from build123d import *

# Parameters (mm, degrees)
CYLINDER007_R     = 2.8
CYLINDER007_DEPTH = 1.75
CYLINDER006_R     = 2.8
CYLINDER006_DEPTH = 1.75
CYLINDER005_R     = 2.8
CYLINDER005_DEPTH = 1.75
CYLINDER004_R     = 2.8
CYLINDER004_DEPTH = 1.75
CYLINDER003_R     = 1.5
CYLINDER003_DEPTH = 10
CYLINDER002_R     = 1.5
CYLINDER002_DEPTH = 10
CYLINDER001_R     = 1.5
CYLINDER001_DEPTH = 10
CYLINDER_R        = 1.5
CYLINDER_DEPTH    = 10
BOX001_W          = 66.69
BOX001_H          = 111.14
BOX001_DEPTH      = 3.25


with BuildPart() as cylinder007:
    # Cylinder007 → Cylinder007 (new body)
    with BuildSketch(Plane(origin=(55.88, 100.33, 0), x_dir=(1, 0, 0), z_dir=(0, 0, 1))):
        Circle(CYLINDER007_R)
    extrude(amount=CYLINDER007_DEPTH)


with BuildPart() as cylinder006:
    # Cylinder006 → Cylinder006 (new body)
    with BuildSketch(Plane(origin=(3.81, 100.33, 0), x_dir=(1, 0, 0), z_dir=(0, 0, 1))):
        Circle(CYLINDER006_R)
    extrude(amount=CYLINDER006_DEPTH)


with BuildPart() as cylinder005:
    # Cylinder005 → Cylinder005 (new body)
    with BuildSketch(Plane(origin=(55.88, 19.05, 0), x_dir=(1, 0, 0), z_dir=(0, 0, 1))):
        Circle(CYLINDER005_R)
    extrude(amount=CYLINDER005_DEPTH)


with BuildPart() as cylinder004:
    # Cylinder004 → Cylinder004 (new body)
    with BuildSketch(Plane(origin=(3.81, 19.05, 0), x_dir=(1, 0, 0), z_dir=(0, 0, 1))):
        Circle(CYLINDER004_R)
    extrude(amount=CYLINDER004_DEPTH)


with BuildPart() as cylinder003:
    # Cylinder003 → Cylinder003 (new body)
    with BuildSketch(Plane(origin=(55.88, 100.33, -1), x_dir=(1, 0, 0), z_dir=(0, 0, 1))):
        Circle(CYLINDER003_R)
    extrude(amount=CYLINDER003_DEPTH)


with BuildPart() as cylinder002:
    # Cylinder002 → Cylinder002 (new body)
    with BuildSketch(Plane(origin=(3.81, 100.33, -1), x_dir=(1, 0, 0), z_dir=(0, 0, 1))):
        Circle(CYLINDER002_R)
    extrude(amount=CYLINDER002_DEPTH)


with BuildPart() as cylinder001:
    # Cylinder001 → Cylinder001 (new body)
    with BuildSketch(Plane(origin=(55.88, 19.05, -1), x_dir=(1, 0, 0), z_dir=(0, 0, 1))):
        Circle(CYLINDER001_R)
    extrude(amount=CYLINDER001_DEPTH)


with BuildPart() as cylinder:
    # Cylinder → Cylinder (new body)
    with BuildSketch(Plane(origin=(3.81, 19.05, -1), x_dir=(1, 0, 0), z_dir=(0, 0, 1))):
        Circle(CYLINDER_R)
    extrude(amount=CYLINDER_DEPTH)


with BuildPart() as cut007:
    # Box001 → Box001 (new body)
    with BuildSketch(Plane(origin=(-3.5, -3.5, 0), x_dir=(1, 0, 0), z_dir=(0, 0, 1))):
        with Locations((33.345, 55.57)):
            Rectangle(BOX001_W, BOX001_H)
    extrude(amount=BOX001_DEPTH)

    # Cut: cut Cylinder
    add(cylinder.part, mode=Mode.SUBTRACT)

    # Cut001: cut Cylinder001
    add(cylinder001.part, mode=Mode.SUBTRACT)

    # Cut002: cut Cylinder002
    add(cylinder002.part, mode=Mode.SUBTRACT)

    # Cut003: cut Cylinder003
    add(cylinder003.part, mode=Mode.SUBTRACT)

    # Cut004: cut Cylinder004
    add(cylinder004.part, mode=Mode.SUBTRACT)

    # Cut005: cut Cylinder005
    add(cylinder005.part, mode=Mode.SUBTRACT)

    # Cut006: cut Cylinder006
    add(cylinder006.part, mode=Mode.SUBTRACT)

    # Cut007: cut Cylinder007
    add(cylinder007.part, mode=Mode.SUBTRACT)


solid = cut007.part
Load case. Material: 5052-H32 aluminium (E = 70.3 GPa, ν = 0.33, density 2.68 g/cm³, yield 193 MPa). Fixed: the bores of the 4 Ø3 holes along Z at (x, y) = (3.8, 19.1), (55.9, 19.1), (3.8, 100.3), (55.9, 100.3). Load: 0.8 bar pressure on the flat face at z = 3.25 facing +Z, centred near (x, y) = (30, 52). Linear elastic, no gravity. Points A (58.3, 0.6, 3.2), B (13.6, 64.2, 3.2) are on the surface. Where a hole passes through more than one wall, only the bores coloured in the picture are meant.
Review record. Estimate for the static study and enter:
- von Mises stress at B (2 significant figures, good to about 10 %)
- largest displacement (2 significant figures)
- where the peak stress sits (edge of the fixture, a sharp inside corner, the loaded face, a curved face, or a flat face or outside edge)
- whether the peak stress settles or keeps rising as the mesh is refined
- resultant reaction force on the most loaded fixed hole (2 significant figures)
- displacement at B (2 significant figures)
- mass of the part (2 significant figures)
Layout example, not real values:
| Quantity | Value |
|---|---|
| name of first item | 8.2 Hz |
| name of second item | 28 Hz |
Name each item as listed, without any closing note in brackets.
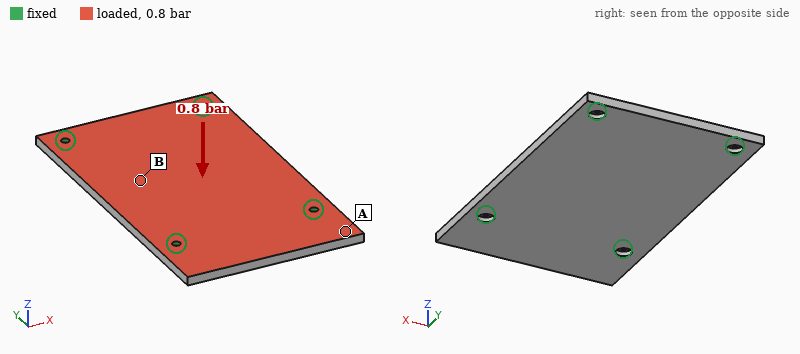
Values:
| Quantity | Value |
|---|---|
| von Mises stress at B | 14 MPa |
| largest displacement | 87 µm |
| where the peak stress sits | edge of the fixture |
| whether the peak stress settles or keeps rising as the mesh is refined | keeps rising |
| resultant reaction force on the most loaded fixed hole | 300 N |
| displacement at B | 83 µm |
| mass of the part | 64 g |
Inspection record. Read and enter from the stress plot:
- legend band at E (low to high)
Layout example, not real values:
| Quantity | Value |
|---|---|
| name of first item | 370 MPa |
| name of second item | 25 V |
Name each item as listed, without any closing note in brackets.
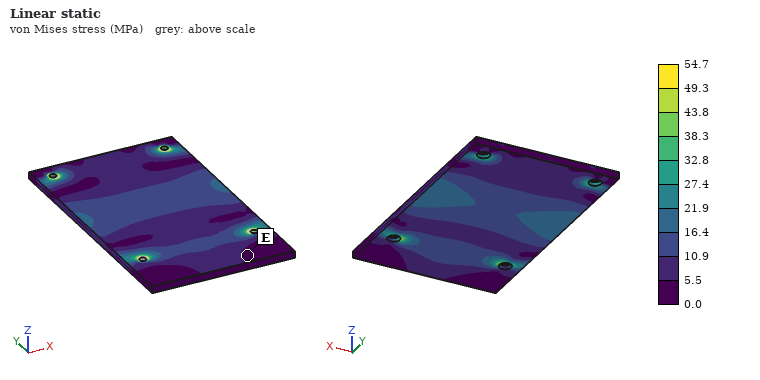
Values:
| Quantity | Value |
|---|---|
| legend band at E | 0.0 to 5.5 MPa |
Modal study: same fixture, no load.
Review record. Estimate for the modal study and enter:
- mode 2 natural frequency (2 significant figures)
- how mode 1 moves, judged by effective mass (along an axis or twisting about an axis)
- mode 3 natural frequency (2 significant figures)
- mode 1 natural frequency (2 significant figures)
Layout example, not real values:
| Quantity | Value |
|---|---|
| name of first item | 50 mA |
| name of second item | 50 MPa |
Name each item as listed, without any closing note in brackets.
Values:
| Quantity | Value |
|---|---|
| mode 2 natural frequency | 2900 Hz |
| how mode 1 moves, judged by effective mass | along Z |
| mode 3 natural frequency | 2900 Hz |
| mode 1 natural frequency | 1800 Hz |
